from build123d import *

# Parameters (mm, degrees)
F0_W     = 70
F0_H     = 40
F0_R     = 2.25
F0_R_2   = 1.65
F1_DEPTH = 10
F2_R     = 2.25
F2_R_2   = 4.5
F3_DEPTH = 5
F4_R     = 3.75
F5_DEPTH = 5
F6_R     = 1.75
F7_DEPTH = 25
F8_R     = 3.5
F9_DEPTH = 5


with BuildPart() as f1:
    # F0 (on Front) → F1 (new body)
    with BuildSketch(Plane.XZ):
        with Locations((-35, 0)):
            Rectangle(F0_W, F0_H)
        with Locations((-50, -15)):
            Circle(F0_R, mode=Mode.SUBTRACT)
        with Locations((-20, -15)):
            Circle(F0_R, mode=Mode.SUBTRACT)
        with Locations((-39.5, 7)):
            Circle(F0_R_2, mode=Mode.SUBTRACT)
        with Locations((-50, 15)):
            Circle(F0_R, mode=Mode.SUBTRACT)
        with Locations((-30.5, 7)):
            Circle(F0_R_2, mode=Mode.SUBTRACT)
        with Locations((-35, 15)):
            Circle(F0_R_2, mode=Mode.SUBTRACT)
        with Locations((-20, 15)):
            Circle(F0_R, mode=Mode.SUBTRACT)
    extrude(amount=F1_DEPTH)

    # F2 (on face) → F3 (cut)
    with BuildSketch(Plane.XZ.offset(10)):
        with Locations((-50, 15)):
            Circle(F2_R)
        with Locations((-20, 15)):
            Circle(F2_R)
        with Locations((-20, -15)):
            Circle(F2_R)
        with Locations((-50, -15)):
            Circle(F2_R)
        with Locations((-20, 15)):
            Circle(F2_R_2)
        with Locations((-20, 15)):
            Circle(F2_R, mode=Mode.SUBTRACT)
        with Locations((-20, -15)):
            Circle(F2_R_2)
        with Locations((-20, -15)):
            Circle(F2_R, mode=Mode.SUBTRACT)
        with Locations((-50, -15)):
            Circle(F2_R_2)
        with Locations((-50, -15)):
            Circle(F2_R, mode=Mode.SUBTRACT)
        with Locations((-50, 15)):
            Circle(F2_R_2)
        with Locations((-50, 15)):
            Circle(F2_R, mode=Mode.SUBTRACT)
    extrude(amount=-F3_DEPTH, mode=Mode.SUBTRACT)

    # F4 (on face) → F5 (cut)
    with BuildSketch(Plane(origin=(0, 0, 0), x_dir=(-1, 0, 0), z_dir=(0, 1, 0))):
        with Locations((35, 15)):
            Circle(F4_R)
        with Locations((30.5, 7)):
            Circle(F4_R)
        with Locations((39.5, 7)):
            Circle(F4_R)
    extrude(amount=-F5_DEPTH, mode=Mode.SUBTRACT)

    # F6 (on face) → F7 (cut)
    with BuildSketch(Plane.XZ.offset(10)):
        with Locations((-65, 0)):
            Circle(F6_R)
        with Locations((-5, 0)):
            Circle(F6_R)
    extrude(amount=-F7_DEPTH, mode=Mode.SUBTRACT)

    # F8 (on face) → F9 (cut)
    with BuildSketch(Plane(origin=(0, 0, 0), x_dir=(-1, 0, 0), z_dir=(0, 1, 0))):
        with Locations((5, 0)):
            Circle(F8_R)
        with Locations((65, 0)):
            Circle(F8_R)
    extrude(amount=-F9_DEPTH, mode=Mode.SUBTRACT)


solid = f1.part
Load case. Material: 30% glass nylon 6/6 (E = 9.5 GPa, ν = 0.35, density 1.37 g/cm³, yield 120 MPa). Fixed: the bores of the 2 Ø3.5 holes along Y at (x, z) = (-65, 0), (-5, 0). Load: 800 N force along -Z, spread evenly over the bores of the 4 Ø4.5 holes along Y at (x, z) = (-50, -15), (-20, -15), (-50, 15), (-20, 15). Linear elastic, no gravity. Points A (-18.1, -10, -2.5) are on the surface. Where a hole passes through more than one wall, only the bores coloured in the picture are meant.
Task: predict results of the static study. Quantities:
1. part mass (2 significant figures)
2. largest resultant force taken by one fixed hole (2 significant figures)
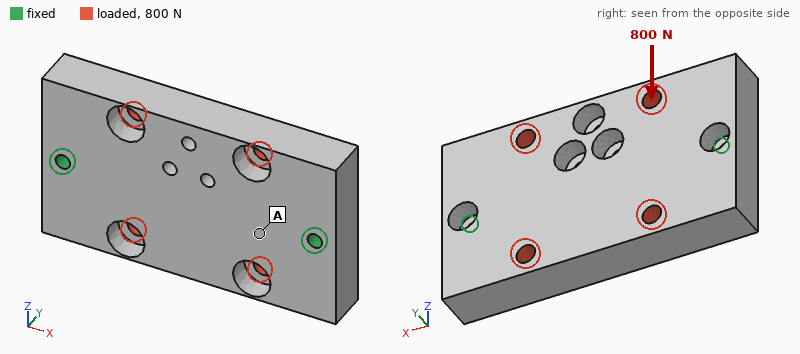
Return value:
34 g
400 N
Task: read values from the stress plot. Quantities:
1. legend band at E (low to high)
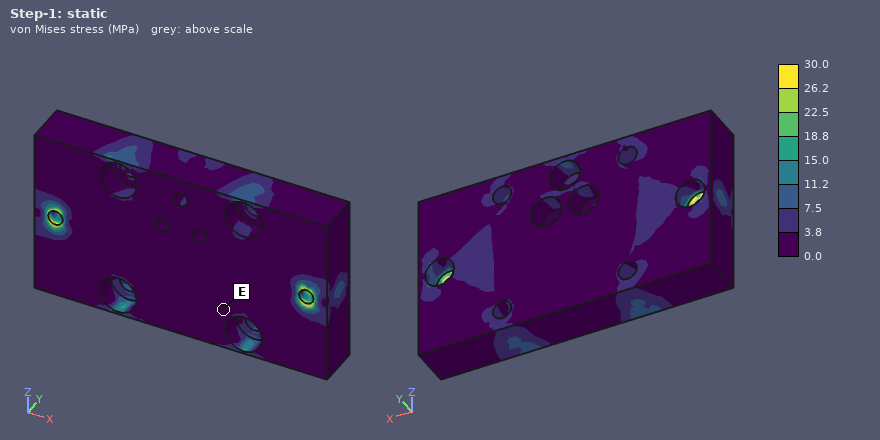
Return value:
0.0 to 3.8 MPa
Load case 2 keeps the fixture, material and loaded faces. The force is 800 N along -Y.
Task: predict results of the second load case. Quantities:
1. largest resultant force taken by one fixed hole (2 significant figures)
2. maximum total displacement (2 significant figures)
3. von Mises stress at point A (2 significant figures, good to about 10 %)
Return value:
540 N
96 µm
4.8 MPa
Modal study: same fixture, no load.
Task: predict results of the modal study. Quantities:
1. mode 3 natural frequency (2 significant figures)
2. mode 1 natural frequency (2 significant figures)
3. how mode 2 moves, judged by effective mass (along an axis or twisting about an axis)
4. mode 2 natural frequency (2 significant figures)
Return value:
5700 Hz
2500 Hz
along Y
3600 Hz
